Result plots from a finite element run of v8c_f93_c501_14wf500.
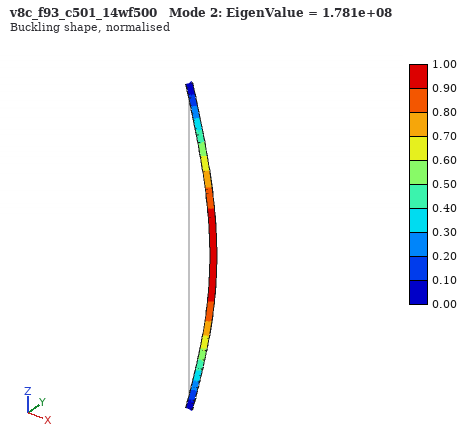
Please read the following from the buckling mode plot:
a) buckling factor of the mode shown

1.781e+08
